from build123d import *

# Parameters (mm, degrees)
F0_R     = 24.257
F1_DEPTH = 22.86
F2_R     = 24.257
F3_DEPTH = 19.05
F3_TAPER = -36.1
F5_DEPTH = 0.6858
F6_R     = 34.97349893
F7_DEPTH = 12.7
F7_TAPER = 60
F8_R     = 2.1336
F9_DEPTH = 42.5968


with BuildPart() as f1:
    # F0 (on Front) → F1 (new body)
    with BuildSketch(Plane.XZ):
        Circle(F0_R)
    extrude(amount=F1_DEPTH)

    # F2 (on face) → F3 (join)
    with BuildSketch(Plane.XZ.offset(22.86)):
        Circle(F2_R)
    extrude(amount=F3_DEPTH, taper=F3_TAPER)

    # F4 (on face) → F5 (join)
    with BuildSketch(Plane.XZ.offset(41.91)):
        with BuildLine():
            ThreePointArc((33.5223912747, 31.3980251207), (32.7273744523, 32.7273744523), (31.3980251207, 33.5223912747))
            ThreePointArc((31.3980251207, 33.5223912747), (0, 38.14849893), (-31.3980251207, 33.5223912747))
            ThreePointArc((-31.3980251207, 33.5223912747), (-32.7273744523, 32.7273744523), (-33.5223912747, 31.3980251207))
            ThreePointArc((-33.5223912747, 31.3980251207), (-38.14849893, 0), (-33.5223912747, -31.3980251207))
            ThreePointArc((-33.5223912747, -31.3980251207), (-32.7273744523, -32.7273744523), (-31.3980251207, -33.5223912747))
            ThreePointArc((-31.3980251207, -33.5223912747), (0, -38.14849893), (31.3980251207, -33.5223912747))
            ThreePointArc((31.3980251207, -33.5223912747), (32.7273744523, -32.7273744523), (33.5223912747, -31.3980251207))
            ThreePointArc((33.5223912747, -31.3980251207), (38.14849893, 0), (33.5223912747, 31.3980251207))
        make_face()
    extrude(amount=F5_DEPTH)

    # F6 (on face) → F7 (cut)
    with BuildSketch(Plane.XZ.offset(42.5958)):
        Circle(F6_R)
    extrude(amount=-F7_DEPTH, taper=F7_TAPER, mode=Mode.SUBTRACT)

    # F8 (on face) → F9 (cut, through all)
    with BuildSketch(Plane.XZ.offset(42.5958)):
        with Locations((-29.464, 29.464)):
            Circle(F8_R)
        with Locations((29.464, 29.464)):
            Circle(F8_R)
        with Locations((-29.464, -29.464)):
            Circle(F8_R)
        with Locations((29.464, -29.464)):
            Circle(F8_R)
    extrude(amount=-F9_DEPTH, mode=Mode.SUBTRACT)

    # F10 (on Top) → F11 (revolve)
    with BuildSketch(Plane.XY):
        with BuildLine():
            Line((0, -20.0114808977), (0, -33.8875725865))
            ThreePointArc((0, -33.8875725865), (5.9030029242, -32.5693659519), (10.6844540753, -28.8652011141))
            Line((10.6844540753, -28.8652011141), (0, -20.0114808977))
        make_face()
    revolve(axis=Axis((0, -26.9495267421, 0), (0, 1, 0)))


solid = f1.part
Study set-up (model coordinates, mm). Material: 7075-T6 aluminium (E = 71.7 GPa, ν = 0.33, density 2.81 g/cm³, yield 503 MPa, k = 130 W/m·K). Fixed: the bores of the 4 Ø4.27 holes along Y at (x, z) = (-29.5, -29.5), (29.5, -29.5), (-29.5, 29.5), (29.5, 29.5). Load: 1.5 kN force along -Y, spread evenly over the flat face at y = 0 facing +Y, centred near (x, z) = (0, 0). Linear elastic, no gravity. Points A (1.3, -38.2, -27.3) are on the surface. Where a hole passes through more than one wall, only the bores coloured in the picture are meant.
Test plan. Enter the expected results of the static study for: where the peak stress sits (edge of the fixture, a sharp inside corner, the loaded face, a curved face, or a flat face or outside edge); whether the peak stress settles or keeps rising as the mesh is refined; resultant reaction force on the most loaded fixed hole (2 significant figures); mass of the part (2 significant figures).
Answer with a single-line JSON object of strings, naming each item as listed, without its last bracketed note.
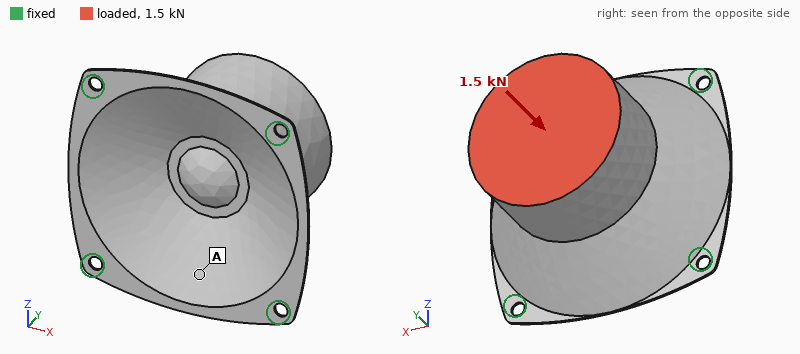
{"where the peak stress sits": "edge of the fixture", "whether the peak stress settles or keeps rising as the mesh is refined": "keeps rising", "resultant reaction force on the most loaded fixed hole": "590 N", "mass of the part": "230 g"}
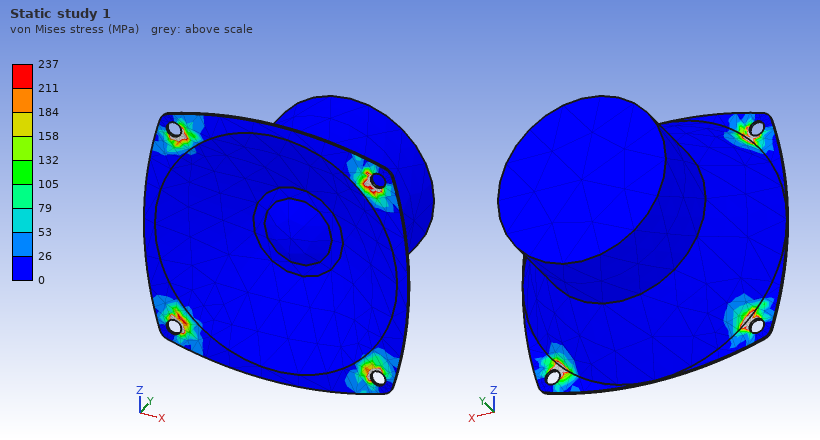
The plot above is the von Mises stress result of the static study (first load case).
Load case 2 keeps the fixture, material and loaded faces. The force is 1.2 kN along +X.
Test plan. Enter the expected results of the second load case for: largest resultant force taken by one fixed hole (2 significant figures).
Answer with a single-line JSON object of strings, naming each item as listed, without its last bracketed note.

{"largest resultant force taken by one fixed hole": "690 N"}
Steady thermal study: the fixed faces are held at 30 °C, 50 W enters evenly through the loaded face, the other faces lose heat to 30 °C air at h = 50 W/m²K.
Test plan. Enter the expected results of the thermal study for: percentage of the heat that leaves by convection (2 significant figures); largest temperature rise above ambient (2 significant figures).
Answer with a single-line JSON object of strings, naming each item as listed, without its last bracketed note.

{"percentage of the heat that leaves by convection": "42 %", "largest temperature rise above ambient": "37 K"}
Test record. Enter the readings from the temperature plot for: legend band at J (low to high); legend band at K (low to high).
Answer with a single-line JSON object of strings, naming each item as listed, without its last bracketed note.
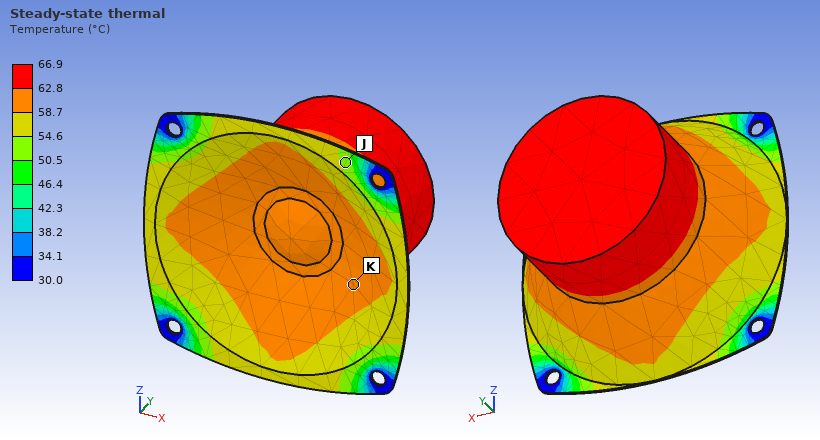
{"legend band at J": "50.5 to 54.6 °C", "legend band at K": "58.7 to 62.8 °C"}
